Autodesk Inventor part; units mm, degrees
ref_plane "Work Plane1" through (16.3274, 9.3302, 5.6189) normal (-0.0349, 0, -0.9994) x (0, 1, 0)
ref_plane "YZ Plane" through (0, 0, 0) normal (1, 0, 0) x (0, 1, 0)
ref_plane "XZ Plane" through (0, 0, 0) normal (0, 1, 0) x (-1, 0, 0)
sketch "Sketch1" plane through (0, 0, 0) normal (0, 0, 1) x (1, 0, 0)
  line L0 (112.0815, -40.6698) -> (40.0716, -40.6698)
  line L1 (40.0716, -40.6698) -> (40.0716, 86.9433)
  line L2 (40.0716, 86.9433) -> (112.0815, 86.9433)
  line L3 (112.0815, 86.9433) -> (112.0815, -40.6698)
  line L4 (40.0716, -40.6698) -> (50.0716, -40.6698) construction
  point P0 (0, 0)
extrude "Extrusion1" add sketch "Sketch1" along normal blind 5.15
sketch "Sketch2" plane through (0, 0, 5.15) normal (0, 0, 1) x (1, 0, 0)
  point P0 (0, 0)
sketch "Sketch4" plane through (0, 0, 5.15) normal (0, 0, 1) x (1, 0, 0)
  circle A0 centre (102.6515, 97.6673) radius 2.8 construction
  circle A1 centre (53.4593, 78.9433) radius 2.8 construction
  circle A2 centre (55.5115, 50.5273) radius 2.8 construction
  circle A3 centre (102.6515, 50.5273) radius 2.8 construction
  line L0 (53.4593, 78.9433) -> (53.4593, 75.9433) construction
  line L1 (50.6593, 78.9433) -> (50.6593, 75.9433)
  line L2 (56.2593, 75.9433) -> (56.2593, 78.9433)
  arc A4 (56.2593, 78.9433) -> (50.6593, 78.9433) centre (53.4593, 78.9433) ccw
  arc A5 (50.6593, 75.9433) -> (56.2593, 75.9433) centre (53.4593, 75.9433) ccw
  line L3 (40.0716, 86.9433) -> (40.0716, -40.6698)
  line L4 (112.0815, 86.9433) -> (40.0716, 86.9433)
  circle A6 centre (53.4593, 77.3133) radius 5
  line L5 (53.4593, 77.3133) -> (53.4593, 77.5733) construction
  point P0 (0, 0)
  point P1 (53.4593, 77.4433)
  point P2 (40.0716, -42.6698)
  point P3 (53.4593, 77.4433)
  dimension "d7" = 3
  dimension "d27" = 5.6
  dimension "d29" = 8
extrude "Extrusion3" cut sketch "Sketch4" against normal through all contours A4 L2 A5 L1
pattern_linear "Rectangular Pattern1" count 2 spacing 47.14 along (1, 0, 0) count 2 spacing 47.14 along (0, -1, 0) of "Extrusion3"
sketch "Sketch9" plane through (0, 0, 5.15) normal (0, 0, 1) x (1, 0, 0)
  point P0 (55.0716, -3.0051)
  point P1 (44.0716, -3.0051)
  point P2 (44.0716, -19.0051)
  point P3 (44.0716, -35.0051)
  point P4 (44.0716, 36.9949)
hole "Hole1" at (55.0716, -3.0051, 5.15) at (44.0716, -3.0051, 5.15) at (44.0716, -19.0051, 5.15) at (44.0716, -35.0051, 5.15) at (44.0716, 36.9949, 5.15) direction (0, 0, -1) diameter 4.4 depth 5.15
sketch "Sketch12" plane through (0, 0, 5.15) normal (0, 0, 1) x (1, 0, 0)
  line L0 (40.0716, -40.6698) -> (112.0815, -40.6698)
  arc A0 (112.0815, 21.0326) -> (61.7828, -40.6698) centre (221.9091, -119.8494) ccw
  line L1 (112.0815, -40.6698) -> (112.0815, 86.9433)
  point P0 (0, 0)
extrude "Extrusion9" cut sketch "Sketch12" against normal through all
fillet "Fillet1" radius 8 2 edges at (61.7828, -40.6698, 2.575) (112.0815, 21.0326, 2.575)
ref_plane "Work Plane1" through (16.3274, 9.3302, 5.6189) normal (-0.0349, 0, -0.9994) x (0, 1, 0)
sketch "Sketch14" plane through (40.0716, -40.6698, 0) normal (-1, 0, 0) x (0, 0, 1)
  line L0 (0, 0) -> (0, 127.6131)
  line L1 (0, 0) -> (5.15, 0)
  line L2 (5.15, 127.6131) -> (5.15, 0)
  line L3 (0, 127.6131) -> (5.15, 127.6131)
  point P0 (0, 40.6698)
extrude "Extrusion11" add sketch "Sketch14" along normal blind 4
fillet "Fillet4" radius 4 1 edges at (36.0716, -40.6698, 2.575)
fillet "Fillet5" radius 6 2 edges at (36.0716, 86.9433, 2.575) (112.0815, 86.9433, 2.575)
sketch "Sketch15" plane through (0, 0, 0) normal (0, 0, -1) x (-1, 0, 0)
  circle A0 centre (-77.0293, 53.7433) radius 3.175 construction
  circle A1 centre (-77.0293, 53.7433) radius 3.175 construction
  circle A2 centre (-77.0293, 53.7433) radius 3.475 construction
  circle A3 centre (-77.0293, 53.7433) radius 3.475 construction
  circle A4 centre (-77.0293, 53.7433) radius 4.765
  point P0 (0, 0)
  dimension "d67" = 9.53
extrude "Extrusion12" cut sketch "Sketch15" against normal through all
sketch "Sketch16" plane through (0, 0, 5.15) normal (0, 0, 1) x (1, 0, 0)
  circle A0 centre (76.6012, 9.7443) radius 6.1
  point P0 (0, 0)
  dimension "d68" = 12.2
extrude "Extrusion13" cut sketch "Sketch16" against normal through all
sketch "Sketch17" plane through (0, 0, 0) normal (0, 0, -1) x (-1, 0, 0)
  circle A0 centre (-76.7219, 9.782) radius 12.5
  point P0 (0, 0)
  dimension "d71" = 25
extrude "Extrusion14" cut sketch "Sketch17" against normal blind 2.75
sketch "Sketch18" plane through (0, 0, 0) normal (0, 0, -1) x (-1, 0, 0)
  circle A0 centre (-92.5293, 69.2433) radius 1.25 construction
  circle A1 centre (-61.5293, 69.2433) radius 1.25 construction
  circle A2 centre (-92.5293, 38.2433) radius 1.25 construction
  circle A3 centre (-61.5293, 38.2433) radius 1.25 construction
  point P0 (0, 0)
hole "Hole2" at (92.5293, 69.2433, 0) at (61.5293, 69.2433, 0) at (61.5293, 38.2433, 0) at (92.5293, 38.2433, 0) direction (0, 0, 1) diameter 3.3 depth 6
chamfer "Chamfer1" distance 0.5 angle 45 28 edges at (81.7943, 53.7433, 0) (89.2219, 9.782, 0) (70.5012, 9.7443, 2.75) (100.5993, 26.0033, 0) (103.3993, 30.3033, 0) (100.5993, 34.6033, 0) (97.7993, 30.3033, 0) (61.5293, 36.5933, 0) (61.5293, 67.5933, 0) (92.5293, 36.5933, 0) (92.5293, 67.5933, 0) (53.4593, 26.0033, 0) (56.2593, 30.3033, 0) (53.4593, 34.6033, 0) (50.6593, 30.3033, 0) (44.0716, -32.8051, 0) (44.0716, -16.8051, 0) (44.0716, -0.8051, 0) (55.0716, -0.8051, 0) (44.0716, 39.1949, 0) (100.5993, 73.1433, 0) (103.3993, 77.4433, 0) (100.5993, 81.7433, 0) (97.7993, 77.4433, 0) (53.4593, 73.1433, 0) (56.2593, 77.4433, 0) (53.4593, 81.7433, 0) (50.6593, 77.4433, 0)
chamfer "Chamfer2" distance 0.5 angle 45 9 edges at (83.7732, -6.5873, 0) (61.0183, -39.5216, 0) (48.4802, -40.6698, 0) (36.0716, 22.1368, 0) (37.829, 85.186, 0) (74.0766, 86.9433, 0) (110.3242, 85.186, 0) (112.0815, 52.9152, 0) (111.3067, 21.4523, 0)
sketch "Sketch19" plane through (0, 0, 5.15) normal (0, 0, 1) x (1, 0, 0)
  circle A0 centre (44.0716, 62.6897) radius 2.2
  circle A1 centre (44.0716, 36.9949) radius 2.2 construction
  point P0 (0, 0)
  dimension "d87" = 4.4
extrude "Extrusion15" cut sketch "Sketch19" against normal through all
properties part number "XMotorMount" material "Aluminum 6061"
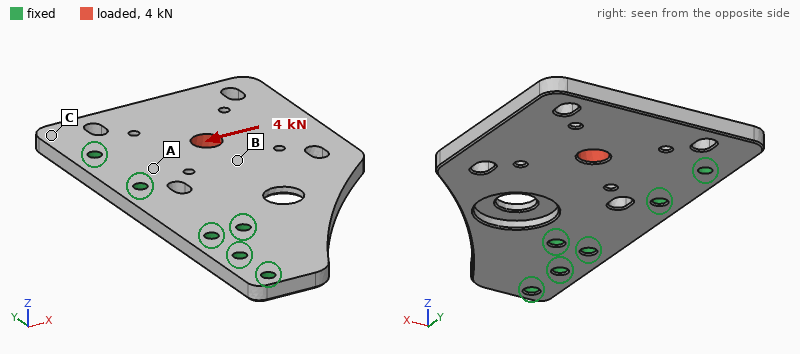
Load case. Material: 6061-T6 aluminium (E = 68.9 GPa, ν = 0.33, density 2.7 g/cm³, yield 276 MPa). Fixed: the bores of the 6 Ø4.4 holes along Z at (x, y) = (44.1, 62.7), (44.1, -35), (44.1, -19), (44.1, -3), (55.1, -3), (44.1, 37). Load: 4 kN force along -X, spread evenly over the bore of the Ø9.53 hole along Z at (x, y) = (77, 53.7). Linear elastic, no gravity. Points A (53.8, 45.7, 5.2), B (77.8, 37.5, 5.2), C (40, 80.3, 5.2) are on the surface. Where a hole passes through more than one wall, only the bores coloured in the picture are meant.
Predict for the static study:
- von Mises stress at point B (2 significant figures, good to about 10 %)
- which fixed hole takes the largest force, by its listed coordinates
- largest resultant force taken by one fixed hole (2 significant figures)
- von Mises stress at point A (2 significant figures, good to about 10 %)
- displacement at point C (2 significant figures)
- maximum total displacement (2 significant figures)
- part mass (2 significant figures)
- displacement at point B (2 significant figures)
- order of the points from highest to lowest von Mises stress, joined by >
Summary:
8.3 MPa
(44.1, 62.7)
2.6 kN
16 MPa
8.6 µm
34 µm
100 g
11 µm
A > B > C
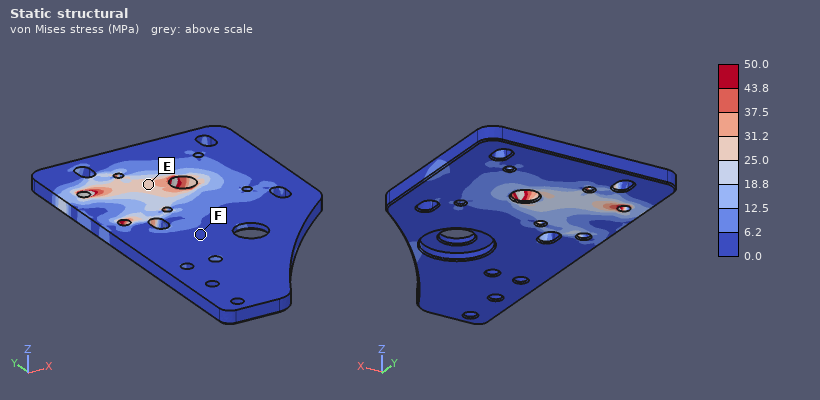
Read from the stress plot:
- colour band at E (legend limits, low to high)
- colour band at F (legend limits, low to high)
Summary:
25.0 to 31.2 MPa
0.0 to 6.2 MPa
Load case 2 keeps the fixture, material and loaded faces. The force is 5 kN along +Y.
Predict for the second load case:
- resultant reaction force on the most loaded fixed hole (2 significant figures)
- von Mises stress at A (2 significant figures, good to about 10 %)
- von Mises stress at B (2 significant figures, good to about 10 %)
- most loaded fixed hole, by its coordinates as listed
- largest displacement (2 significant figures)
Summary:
2.6 kN
26 MPa
27 MPa
(44.1, 62.7)
34 µm
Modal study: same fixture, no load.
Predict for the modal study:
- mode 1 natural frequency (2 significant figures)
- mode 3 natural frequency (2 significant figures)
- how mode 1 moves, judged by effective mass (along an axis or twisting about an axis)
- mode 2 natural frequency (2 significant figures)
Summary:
960 Hz
4800 Hz
along Z
2300 Hz
